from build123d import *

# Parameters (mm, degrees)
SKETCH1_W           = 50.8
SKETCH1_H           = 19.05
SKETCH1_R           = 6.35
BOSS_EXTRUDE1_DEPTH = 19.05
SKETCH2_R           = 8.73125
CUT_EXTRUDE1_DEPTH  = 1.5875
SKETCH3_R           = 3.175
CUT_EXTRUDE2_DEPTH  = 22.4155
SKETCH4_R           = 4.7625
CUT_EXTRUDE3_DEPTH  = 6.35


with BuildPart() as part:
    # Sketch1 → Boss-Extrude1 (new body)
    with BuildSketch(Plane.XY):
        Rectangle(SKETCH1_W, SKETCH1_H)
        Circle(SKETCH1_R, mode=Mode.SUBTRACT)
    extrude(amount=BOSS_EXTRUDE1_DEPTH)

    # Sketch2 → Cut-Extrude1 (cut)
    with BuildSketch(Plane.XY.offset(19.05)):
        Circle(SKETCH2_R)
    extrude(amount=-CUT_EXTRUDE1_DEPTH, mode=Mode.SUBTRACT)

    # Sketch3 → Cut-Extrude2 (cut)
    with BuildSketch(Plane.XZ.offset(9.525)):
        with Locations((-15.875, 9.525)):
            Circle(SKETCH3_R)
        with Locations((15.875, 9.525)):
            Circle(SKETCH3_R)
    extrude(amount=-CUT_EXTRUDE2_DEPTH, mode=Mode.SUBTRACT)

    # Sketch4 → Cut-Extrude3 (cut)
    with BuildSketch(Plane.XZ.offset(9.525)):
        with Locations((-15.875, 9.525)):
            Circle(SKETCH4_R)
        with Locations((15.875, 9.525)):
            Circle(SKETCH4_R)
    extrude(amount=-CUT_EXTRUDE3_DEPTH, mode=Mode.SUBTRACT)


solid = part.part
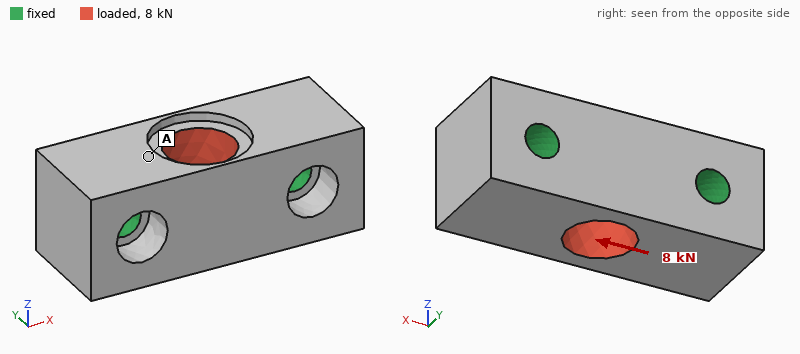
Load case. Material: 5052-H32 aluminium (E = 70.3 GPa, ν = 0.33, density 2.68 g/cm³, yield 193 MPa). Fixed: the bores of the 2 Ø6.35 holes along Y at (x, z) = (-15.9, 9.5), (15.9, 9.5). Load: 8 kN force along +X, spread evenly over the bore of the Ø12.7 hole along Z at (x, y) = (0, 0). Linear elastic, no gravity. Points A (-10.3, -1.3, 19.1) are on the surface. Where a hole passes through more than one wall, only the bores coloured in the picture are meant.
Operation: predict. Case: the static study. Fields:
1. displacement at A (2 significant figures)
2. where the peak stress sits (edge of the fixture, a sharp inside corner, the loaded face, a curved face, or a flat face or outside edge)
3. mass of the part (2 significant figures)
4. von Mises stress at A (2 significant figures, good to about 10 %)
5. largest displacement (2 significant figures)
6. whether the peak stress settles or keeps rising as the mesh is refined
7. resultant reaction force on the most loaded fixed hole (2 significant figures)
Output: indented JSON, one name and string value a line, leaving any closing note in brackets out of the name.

{
  "displacement at A": "2.1 µm",
  "where the peak stress sits": "edge of the fixture",
  "mass of the part": "38 g",
  "von Mises stress at A": "5.5 MPa",
  "largest displacement": "5.8 µm",
  "whether the peak stress settles or keeps rising as the mesh is refined": "keeps rising",
  "resultant reaction force on the most loaded fixed hole": "4.0 kN"
}
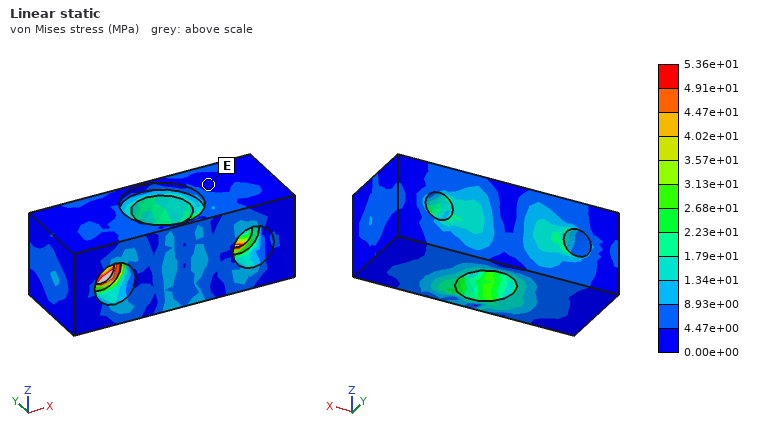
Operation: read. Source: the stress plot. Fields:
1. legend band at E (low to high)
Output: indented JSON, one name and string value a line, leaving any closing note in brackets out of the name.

{
  "legend band at E": "0.00e+00 to 4.47e+00 MPa"
}
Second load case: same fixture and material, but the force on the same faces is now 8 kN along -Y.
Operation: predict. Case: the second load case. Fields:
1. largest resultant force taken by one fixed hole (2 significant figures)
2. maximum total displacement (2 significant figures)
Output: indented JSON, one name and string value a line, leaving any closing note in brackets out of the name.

{
  "largest resultant force taken by one fixed hole": "4.0 kN",
  "maximum total displacement": "13 µm"
}
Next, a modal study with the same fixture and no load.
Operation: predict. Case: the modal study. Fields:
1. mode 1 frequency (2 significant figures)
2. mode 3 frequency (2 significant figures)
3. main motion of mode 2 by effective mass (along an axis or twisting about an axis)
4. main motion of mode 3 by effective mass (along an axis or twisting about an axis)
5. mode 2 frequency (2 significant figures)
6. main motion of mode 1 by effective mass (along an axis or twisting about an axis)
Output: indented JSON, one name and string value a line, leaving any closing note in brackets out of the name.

{
  "mode 1 frequency": "31 kHz",
  "mode 3 frequency": "40 kHz",
  "main motion of mode 2 by effective mass": "twisting about X",
  "main motion of mode 3 by effective mass": "twisting about Y",
  "mode 2 frequency": "37 kHz",
  "main motion of mode 1 by effective mass": "along Z"
}
